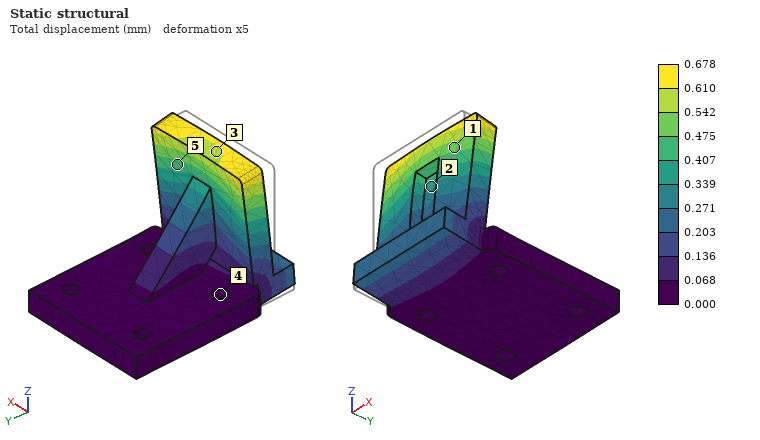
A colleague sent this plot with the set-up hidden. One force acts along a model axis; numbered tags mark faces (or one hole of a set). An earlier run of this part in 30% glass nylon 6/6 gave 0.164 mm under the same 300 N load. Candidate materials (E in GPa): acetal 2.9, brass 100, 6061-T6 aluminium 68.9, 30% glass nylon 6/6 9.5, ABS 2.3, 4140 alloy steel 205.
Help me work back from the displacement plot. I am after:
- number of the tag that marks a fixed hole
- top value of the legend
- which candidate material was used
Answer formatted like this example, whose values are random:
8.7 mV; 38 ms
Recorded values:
4; 0.678 mm; ABS
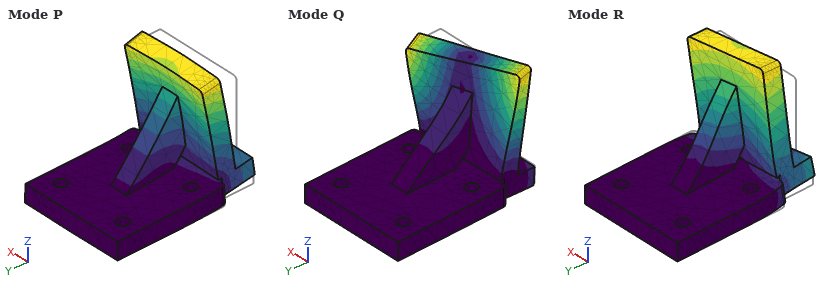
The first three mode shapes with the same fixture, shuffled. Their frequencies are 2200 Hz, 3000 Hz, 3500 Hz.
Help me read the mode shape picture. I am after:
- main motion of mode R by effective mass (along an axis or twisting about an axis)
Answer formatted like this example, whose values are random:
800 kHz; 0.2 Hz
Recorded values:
along X
